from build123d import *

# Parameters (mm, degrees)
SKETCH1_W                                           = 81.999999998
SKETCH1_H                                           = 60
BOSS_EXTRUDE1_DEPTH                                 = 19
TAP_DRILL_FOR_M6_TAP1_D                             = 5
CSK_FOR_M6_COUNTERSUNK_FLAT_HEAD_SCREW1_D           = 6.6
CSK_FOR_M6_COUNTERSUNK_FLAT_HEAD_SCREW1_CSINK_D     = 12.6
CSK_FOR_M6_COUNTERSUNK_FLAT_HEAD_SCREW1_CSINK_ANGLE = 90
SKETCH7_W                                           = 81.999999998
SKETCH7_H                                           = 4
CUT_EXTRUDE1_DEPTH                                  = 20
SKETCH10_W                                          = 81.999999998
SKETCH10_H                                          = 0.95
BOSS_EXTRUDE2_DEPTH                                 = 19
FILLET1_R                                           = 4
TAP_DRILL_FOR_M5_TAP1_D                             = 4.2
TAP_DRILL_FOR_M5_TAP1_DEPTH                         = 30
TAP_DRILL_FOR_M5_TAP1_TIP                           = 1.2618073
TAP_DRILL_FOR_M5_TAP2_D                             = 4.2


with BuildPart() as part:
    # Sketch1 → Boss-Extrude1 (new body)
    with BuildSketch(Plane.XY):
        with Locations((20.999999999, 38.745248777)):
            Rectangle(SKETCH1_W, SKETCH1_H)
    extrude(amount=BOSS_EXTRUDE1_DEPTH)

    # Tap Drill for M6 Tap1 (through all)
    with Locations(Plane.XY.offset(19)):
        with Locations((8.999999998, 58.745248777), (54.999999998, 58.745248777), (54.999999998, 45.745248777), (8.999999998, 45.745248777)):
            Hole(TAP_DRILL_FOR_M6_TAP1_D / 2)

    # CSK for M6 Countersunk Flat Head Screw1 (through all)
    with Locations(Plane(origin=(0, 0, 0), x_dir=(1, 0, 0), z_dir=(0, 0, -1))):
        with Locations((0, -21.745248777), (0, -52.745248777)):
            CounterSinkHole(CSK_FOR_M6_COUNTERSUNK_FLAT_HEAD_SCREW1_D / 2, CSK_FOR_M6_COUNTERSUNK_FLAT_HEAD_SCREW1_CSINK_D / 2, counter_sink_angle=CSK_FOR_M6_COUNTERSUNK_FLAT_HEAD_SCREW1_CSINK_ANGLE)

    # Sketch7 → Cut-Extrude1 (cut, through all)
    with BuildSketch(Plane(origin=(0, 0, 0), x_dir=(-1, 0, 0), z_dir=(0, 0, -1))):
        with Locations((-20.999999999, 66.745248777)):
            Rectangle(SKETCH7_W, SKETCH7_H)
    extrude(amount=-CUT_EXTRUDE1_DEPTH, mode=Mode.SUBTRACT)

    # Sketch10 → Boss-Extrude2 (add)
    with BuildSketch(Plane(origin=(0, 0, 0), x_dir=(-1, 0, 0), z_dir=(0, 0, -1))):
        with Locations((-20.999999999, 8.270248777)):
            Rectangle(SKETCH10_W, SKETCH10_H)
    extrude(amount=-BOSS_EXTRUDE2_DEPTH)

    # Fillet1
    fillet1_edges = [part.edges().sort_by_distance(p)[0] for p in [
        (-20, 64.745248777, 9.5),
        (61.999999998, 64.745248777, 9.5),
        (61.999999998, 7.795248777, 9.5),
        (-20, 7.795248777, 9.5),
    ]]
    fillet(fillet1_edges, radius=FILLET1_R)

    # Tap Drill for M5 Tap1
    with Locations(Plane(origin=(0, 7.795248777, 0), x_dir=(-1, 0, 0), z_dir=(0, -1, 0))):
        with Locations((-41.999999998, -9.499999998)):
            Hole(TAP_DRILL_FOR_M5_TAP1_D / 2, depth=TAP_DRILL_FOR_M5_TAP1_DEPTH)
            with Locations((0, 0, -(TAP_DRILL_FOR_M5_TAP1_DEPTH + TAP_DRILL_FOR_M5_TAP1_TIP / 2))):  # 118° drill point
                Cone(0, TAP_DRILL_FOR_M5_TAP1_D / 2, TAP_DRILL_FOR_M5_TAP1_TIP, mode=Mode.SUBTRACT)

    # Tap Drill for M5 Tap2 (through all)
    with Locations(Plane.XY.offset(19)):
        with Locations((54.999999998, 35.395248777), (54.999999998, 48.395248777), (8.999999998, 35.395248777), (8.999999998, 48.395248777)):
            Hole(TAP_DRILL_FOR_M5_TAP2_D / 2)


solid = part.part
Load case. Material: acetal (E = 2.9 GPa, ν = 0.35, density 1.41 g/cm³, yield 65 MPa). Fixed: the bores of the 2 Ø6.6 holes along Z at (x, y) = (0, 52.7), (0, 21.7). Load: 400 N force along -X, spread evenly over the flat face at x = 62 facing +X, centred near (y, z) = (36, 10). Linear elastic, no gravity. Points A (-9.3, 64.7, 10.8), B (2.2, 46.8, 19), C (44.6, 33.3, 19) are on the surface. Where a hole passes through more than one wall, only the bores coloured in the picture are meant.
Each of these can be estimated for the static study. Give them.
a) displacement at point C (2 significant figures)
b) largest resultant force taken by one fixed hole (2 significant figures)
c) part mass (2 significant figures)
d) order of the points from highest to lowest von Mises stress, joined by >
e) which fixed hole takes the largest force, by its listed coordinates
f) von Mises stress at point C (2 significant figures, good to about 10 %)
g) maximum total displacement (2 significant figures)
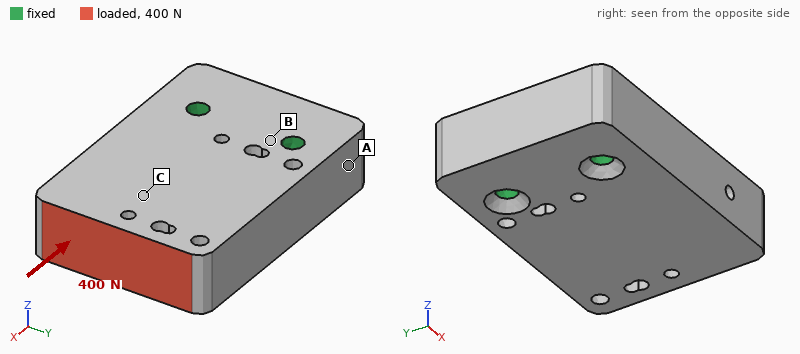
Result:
7.0 µm
210 N
120 g
C > B > A
(0, 21.7)
0.46 MPa
13 µm
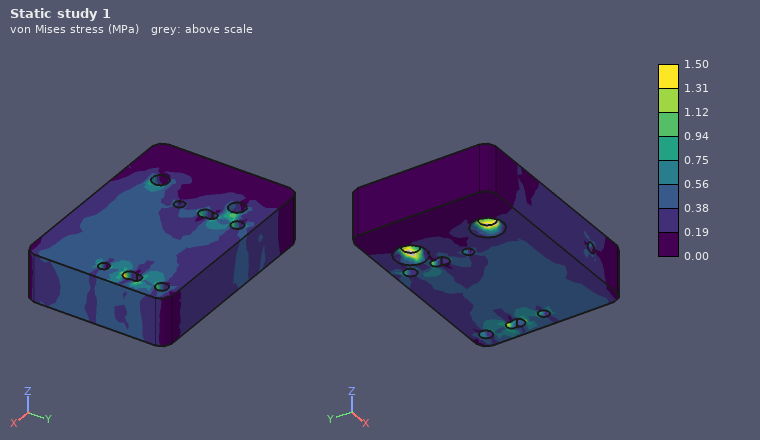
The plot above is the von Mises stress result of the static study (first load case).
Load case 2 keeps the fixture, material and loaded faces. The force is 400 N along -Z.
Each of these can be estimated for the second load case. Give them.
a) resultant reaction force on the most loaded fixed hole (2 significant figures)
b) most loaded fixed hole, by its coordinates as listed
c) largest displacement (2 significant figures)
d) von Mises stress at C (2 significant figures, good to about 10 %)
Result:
230 N
(0, 21.7)
0.49 mm
2.2 MPa
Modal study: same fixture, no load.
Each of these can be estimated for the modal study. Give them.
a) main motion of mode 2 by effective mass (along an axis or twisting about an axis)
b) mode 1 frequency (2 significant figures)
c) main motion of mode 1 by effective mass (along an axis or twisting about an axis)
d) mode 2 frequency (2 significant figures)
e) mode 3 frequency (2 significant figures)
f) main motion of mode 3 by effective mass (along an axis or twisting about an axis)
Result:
along Y
940 Hz
along Z
2000 Hz
2200 Hz
twisting about X
